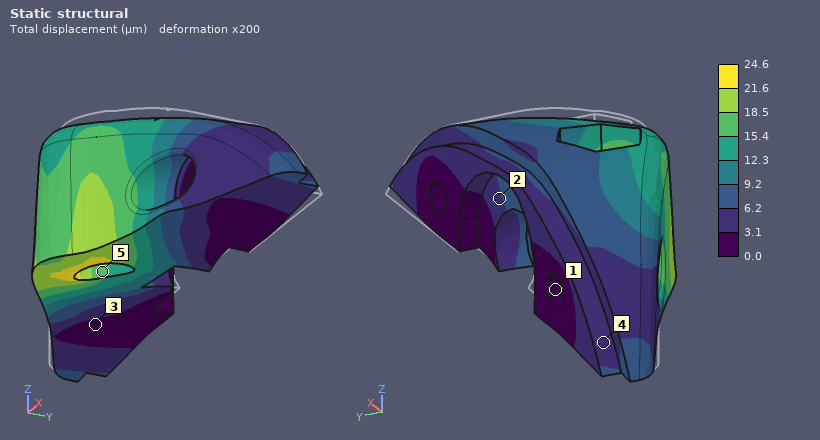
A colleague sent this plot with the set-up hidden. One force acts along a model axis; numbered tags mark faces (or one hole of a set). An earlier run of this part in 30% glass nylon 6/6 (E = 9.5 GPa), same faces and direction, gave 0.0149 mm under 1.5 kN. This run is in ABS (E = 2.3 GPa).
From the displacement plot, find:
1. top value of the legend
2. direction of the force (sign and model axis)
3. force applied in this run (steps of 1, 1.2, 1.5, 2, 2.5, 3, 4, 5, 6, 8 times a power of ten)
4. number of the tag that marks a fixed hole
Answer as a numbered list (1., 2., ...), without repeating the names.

1. 24.6 µm
2. -X
3. 600 N
4. 1
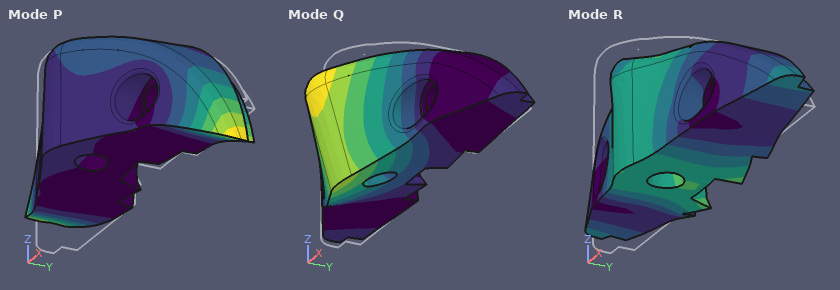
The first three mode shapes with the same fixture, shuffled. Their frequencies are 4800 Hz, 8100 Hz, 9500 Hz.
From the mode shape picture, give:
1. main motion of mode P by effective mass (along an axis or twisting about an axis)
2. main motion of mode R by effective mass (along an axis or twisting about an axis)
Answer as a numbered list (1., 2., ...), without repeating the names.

1. along X
2. along Y
